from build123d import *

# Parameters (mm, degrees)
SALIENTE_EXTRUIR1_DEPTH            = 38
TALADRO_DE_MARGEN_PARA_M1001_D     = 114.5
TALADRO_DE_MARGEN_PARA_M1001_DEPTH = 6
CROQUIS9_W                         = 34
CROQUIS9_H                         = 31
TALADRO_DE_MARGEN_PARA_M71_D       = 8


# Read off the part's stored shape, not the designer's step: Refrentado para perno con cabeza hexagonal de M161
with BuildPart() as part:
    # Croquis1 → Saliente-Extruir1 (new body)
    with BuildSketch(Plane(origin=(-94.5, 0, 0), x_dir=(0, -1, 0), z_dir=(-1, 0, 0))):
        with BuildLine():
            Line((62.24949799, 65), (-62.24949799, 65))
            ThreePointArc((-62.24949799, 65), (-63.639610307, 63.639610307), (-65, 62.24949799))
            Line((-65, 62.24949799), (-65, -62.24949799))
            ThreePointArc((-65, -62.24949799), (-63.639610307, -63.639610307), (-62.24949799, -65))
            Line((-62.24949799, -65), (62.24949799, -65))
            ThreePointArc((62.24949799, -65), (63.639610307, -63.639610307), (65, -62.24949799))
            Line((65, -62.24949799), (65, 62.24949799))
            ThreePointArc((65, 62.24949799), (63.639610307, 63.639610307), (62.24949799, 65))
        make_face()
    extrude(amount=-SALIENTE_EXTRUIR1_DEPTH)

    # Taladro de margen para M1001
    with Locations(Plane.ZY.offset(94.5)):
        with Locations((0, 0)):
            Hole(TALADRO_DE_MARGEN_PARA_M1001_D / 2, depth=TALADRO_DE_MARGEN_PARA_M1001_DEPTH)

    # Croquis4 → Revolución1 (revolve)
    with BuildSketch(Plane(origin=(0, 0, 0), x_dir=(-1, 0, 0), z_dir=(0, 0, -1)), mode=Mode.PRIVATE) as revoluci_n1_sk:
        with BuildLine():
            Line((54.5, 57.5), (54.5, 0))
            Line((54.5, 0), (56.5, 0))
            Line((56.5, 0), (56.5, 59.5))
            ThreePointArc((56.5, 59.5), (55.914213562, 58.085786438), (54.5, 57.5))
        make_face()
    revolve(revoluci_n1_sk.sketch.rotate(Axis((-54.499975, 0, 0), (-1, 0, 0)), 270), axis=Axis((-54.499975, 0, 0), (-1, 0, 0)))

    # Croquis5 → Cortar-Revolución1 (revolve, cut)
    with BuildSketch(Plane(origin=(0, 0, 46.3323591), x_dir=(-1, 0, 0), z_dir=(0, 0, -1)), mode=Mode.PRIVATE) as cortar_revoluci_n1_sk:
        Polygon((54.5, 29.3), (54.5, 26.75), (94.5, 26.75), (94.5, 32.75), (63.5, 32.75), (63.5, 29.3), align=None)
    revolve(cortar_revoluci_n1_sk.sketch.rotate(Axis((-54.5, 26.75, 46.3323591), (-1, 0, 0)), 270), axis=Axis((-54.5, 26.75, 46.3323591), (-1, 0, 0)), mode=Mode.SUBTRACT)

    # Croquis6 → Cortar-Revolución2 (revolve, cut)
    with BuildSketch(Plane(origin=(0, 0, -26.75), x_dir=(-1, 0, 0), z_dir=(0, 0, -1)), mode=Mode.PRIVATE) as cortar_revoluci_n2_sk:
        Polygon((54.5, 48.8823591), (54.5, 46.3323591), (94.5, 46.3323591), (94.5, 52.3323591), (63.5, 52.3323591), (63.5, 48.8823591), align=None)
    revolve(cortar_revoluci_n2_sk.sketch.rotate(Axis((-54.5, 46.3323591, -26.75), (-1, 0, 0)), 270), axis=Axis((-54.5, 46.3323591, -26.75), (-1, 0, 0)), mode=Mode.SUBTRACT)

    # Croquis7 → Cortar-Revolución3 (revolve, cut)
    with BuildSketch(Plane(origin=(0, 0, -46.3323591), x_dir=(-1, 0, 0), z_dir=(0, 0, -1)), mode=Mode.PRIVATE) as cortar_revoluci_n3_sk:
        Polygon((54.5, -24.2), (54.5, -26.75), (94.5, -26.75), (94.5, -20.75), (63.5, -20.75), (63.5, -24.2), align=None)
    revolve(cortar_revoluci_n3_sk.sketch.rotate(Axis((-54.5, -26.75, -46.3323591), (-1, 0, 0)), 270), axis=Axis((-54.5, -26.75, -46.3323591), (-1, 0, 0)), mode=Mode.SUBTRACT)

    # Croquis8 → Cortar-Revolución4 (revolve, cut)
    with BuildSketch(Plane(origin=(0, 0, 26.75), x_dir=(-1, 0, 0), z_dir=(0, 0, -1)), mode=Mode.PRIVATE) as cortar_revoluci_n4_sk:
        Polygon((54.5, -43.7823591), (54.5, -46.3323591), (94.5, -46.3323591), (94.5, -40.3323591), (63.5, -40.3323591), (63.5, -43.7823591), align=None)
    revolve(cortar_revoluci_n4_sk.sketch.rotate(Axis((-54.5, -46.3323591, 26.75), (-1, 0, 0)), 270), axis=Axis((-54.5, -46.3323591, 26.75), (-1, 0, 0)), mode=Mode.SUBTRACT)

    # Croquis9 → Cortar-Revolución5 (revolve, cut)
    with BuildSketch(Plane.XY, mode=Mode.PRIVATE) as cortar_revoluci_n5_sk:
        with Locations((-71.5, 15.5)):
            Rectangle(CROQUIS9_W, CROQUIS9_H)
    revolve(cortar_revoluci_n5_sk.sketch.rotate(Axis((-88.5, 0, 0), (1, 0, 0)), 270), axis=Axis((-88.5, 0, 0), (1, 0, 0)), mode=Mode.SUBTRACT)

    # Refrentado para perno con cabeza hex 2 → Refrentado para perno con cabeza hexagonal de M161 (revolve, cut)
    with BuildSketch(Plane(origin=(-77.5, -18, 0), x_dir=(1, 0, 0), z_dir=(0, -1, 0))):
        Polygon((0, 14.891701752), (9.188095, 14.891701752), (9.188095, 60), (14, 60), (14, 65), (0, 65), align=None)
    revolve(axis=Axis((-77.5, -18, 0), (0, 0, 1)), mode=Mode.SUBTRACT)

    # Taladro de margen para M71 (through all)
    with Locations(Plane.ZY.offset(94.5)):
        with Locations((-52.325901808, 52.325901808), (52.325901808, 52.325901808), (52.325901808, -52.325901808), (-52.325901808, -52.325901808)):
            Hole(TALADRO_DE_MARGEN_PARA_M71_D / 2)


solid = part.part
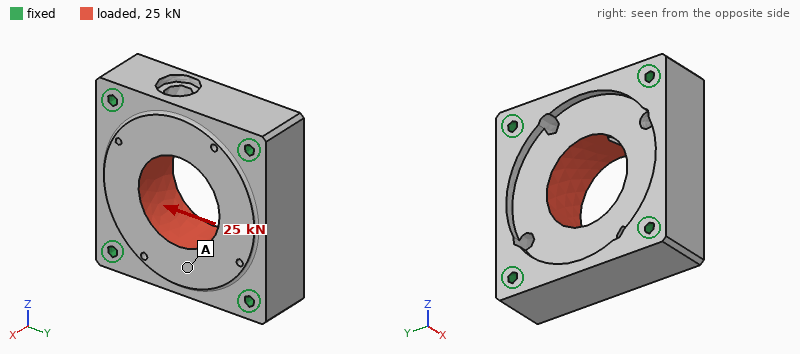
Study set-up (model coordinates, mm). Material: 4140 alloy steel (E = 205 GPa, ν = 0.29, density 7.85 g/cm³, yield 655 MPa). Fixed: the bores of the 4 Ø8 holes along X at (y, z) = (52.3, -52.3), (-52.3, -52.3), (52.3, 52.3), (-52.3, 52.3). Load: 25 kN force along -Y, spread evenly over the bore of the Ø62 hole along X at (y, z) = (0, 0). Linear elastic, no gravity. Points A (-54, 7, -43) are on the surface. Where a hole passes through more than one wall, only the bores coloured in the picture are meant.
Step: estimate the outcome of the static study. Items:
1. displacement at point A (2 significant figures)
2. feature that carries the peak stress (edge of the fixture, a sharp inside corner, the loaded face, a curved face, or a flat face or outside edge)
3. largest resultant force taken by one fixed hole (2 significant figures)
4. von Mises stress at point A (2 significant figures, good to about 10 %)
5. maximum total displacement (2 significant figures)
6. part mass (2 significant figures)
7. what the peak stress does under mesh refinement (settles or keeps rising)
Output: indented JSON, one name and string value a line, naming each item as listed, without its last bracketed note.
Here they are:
{
  "displacement at point A": "1.2 µm",
  "feature that carries the peak stress": "edge of the fixture",
  "largest resultant force taken by one fixed hole": "7.4 kN",
  "von Mises stress at point A": "5.9 MPa",
  "maximum total displacement": "3.2 µm",
  "part mass": "3.7 kg",
  "what the peak stress does under mesh refinement": "keeps rising"
}
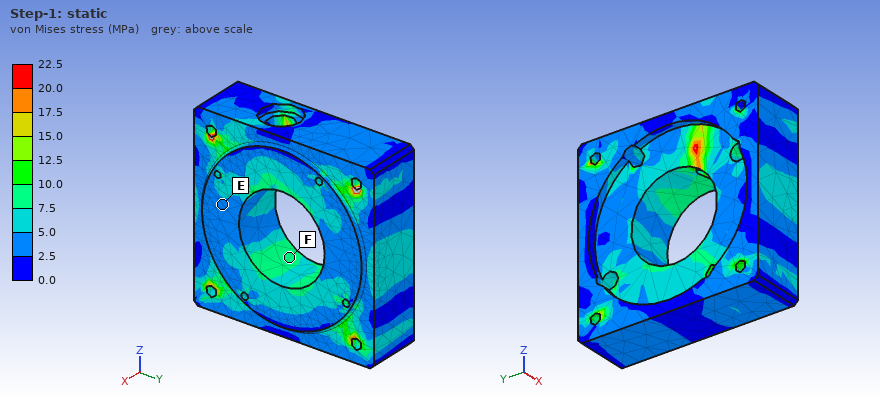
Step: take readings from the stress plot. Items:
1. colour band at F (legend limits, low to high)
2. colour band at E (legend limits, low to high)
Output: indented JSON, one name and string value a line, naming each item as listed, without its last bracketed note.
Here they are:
{
  "colour band at F": "7.5 to 10.0 MPa",
  "colour band at E": "2.5 to 5.0 MPa"
}
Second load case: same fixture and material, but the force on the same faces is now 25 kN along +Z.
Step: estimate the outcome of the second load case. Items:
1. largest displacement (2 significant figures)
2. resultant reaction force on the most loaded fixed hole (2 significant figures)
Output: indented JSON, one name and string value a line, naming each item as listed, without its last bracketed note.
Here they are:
{
  "largest displacement": "3.0 µm",
  "resultant reaction force on the most loaded fixed hole": "7.2 kN"
}
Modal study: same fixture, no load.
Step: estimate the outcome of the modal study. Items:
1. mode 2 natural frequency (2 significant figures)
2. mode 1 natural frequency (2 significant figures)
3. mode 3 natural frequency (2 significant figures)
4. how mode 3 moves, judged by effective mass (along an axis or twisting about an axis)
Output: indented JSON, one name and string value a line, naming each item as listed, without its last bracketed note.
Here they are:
{
  "mode 2 natural frequency": "8700 Hz",
  "mode 1 natural frequency": "8400 Hz",
  "mode 3 natural frequency": "11 kHz",
  "how mode 3 moves, judged by effective mass": "twisting about Y"
}
